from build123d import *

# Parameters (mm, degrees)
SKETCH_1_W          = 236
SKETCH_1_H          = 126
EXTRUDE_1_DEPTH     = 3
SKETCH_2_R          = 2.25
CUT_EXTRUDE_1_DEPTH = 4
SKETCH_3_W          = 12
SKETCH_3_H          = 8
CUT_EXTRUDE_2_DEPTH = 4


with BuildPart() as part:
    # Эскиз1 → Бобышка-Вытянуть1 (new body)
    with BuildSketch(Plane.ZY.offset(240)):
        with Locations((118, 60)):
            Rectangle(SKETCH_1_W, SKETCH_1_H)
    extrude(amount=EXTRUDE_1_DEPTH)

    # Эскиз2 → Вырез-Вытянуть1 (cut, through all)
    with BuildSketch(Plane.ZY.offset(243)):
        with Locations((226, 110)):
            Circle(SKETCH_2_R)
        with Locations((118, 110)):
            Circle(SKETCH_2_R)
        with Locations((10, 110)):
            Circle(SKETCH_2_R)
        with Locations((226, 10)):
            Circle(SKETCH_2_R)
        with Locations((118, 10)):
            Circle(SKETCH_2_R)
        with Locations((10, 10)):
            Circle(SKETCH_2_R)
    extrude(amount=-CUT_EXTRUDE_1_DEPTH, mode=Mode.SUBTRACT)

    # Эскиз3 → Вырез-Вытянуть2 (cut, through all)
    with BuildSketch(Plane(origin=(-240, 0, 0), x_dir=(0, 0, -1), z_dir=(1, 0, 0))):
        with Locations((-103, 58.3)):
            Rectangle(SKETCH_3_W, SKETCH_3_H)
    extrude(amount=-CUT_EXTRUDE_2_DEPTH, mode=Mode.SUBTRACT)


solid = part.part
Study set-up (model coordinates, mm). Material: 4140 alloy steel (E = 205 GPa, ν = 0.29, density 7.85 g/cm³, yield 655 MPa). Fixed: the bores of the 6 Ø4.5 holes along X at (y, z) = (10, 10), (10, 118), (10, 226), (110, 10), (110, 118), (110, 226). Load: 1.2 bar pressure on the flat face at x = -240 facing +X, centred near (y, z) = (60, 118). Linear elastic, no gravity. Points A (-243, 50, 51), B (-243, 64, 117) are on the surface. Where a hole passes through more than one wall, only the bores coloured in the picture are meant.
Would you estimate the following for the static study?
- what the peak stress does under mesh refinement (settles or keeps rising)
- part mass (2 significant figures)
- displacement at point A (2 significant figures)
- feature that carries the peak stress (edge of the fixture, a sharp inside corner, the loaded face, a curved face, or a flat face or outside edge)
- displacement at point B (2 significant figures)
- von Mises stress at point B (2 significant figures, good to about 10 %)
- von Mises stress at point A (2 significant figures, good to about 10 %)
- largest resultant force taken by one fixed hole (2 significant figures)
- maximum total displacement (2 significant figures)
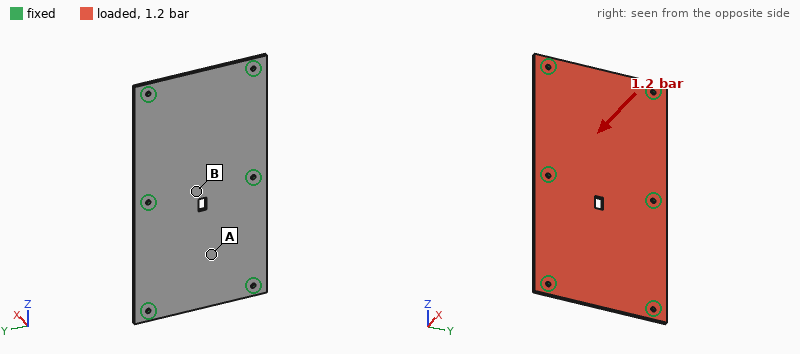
keeps rising
700 g
0.19 mm
edge of the fixture
0.14 mm
66 MPa
40 MPa
850 N
0.20 mm
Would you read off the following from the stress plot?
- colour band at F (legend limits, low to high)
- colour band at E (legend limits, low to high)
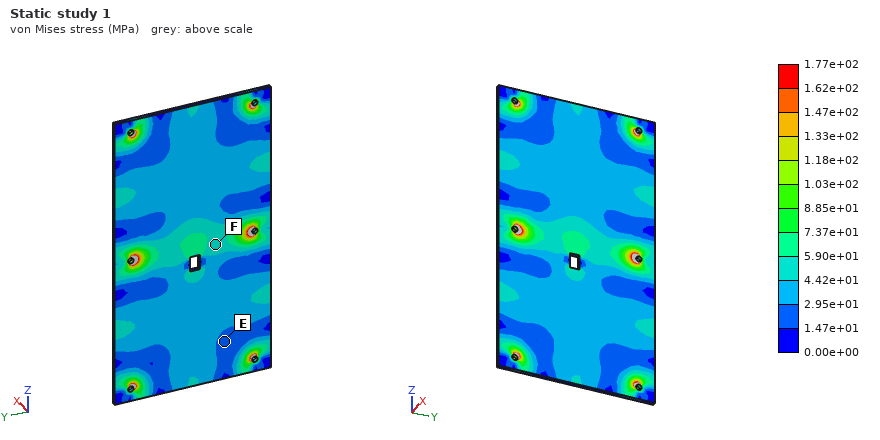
4.42e+01 to 5.90e+01 MPa
1.47e+01 to 2.95e+01 MPa
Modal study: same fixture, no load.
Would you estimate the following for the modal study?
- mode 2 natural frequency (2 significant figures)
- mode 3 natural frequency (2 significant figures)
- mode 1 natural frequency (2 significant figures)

970 Hz
1500 Hz
960 Hz
